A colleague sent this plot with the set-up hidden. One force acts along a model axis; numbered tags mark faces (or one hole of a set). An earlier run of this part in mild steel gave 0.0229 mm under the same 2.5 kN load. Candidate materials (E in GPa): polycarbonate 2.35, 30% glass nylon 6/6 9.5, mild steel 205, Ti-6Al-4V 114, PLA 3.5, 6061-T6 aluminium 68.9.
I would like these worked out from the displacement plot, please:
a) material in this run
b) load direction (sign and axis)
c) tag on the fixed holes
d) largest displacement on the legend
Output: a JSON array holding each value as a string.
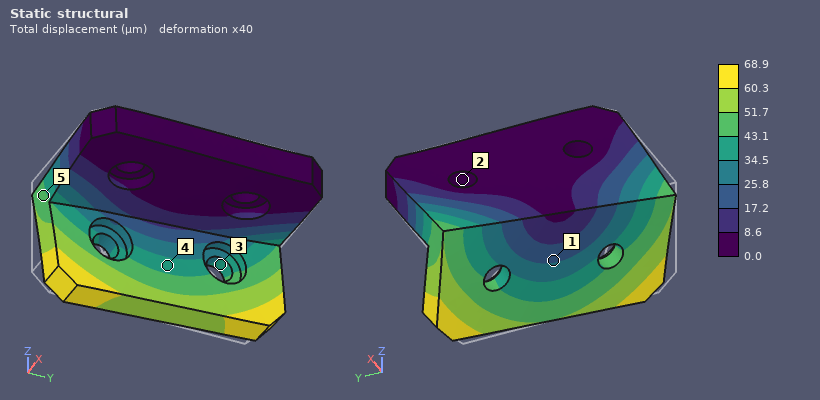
["6061-T6 aluminium", "+Y", "2", "68.9 µm"]
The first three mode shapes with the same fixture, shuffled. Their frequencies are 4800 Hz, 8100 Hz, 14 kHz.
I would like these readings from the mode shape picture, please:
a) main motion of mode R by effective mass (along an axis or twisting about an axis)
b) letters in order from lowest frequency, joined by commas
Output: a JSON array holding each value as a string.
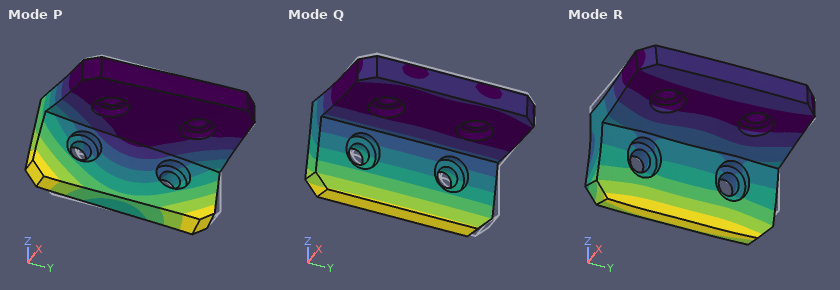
["along Z", "Q, P, R"]
